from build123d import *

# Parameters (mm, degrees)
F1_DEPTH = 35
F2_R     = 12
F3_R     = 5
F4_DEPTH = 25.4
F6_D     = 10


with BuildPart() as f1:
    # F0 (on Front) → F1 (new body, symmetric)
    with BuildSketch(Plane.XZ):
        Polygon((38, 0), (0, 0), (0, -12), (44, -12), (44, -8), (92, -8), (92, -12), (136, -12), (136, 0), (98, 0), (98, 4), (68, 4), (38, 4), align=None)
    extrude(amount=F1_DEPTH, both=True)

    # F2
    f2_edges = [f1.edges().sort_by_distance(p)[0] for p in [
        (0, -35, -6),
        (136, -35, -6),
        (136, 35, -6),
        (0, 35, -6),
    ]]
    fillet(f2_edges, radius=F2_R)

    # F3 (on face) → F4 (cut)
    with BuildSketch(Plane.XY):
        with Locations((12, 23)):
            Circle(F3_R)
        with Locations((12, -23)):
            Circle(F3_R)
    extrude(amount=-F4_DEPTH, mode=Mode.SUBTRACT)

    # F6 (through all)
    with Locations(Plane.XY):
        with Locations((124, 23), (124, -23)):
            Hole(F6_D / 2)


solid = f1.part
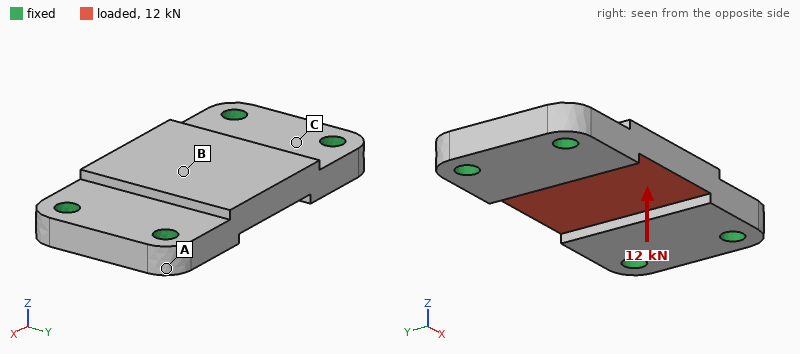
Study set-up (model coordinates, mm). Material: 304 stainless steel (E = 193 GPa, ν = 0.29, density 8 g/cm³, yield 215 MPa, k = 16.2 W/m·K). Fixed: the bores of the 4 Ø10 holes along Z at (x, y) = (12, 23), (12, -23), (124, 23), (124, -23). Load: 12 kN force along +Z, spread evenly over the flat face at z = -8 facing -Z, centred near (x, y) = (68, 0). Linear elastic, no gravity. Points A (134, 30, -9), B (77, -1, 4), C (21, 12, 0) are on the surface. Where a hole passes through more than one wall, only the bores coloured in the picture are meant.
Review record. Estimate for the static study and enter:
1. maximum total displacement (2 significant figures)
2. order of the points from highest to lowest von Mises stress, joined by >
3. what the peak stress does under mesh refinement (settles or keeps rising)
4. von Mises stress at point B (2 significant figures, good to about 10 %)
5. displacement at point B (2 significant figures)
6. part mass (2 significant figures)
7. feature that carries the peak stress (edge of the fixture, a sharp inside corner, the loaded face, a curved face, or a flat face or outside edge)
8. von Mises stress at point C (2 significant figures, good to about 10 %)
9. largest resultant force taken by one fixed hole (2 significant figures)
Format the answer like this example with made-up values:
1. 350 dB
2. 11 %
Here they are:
1. 36 µm
2. B > C > A
3. keeps rising
4. 48 MPa
5. 32 µm
6. 900 g
7. edge of the fixture
8. 30 MPa
9. 5.2 kN
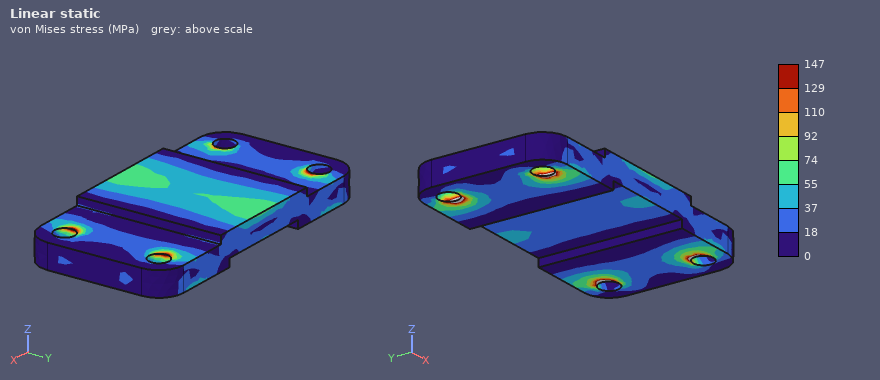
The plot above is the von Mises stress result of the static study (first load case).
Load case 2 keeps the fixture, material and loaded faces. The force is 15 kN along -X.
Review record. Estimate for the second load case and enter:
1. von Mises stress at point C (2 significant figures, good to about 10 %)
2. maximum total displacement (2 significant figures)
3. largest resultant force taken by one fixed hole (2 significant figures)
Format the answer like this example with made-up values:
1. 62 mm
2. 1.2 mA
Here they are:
1. 12 MPa
2. 3.6 µm
3. 3.8 kN
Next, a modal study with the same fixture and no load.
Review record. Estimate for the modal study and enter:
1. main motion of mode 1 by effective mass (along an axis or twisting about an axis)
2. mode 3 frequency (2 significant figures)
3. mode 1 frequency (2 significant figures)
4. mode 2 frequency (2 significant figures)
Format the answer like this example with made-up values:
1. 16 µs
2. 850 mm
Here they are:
1. along Z
2. 11 kHz
3. 4900 Hz
4. 6800 Hz
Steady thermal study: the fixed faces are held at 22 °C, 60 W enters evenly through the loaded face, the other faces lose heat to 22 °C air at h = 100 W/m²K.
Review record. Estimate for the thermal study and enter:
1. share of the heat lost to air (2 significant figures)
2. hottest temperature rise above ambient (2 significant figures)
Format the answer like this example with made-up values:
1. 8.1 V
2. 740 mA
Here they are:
1. 64 %
2. 57 K
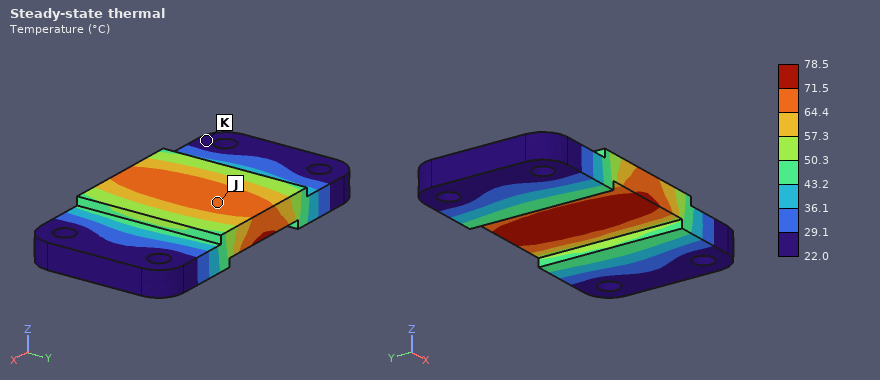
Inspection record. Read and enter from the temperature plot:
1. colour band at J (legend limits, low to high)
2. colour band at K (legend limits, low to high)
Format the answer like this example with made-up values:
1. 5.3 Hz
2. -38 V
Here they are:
1. 64.4 to 71.5 °C
2. 22.0 to 29.1 °C
